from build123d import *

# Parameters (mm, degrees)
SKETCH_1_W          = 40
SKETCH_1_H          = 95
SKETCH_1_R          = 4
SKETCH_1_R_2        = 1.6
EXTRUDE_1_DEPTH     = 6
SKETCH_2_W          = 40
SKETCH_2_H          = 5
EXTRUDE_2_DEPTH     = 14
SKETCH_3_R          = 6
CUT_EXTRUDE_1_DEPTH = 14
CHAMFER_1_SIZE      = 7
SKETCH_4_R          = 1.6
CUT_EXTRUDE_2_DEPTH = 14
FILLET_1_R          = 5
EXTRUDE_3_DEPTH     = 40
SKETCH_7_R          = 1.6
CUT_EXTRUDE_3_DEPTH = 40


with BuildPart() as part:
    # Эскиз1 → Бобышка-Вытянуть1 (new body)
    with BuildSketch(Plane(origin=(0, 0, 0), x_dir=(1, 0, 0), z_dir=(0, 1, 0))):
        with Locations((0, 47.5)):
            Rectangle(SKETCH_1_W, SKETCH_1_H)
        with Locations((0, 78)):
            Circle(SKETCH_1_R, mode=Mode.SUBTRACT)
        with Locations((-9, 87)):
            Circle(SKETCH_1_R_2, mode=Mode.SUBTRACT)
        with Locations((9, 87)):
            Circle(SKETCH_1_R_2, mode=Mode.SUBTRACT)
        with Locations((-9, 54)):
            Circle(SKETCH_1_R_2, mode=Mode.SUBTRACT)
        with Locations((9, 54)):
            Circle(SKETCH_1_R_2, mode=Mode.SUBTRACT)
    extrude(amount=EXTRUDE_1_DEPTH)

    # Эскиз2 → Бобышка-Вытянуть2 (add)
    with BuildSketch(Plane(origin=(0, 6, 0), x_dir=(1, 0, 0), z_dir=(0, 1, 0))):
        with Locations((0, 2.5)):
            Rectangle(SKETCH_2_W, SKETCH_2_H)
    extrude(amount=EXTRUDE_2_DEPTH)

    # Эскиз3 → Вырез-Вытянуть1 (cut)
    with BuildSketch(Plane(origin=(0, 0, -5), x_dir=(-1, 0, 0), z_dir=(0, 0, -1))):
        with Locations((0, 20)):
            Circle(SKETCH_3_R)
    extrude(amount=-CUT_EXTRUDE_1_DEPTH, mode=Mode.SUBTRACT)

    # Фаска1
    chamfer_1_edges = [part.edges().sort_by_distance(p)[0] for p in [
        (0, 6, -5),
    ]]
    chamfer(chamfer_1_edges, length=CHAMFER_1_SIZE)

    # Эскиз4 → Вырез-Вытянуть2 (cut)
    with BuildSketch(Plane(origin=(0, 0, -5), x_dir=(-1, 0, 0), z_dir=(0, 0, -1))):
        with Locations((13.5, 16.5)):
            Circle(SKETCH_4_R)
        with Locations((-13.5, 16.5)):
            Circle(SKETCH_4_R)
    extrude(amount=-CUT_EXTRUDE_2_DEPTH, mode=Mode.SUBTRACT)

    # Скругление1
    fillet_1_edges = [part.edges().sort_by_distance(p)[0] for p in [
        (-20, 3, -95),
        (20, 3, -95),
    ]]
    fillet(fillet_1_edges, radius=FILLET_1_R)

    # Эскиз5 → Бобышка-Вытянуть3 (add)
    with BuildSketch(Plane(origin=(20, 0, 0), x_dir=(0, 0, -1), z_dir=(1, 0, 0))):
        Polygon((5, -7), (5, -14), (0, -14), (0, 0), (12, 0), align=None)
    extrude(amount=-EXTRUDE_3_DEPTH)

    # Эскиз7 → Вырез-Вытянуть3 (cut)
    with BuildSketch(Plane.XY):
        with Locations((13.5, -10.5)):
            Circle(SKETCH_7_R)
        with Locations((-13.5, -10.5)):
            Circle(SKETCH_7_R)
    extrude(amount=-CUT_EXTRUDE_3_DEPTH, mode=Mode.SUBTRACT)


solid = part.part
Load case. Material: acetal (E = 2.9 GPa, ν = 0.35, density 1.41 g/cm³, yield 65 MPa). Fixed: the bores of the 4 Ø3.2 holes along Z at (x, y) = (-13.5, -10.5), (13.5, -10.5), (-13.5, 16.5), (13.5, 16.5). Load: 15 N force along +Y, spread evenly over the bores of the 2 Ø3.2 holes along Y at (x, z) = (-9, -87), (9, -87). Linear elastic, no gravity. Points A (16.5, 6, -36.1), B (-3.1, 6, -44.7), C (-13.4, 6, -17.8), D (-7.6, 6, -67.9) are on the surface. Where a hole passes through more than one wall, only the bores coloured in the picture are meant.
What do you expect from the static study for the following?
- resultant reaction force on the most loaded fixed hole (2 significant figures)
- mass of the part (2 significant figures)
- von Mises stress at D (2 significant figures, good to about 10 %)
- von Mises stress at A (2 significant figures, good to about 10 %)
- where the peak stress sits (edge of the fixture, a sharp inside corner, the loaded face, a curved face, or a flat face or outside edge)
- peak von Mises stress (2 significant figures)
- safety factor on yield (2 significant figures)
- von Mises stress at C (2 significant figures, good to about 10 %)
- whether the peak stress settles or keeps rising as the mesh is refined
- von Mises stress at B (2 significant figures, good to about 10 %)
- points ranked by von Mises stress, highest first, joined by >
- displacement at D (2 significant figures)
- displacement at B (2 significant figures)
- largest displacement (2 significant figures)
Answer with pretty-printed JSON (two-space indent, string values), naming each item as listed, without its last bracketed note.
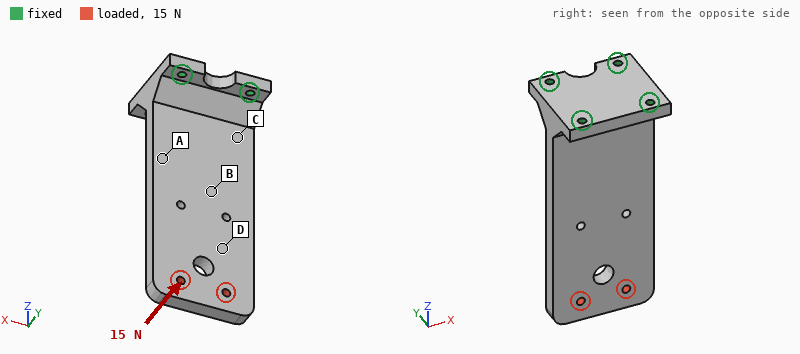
{
  "resultant reaction force on the most loaded fixed hole": "28 N",
  "mass of the part": "41 g",
  "von Mises stress at D": "1.3 MPa",
  "von Mises stress at A": "3.2 MPa",
  "where the peak stress sits": "a curved face",
  "peak von Mises stress": "4.5 MPa",
  "safety factor on yield": "14",
  "von Mises stress at C": "4.0 MPa",
  "whether the peak stress settles or keeps rising as the mesh is refined": "settles",
  "von Mises stress at B": "2.6 MPa",
  "points ranked by von Mises stress, highest first, joined by >": "C > A > B > D",
  "displacement at D": "0.71 mm",
  "displacement at B": "0.30 mm",
  "largest displacement": "1.3 mm"
}
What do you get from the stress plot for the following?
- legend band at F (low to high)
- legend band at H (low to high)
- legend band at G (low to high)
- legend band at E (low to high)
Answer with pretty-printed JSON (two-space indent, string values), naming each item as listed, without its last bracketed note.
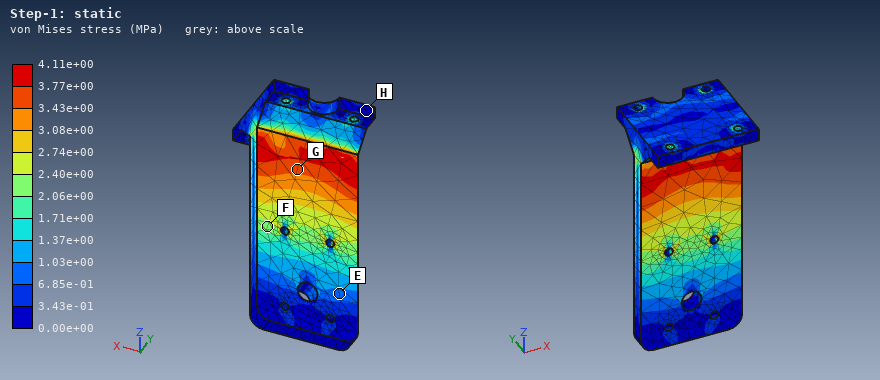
{
  "legend band at F": "2.06e+00 to 2.40e+00 MPa",
  "legend band at H": "0.00e+00 to 3.43e-01 MPa",
  "legend band at G": "3.43e+00 to 3.77e+00 MPa",
  "legend band at E": "6.85e-01 to 1.03e+00 MPa"
}
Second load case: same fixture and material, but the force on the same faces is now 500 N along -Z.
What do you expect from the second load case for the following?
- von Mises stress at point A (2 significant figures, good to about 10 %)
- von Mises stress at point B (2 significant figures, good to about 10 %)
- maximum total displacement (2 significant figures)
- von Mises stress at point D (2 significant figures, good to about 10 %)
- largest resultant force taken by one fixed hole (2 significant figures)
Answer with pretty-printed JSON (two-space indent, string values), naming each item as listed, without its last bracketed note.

{
  "von Mises stress at point A": "2.1 MPa",
  "von Mises stress at point B": "2.1 MPa",
  "maximum total displacement": "94 µm",
  "von Mises stress at point D": "2.5 MPa",
  "largest resultant force taken by one fixed hole": "140 N"
}
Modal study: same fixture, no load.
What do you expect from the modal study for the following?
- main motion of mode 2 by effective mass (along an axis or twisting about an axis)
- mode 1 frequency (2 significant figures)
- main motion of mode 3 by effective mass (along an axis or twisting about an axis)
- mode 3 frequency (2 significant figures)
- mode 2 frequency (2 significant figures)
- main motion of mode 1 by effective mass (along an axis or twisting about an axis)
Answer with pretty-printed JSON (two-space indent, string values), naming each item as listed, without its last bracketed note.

{
  "main motion of mode 2 by effective mass": "along X",
  "mode 1 frequency": "200 Hz",
  "main motion of mode 3 by effective mass": "twisting about Z",
  "mode 3 frequency": "810 Hz",
  "mode 2 frequency": "750 Hz",
  "main motion of mode 1 by effective mass": "along Y"
}
